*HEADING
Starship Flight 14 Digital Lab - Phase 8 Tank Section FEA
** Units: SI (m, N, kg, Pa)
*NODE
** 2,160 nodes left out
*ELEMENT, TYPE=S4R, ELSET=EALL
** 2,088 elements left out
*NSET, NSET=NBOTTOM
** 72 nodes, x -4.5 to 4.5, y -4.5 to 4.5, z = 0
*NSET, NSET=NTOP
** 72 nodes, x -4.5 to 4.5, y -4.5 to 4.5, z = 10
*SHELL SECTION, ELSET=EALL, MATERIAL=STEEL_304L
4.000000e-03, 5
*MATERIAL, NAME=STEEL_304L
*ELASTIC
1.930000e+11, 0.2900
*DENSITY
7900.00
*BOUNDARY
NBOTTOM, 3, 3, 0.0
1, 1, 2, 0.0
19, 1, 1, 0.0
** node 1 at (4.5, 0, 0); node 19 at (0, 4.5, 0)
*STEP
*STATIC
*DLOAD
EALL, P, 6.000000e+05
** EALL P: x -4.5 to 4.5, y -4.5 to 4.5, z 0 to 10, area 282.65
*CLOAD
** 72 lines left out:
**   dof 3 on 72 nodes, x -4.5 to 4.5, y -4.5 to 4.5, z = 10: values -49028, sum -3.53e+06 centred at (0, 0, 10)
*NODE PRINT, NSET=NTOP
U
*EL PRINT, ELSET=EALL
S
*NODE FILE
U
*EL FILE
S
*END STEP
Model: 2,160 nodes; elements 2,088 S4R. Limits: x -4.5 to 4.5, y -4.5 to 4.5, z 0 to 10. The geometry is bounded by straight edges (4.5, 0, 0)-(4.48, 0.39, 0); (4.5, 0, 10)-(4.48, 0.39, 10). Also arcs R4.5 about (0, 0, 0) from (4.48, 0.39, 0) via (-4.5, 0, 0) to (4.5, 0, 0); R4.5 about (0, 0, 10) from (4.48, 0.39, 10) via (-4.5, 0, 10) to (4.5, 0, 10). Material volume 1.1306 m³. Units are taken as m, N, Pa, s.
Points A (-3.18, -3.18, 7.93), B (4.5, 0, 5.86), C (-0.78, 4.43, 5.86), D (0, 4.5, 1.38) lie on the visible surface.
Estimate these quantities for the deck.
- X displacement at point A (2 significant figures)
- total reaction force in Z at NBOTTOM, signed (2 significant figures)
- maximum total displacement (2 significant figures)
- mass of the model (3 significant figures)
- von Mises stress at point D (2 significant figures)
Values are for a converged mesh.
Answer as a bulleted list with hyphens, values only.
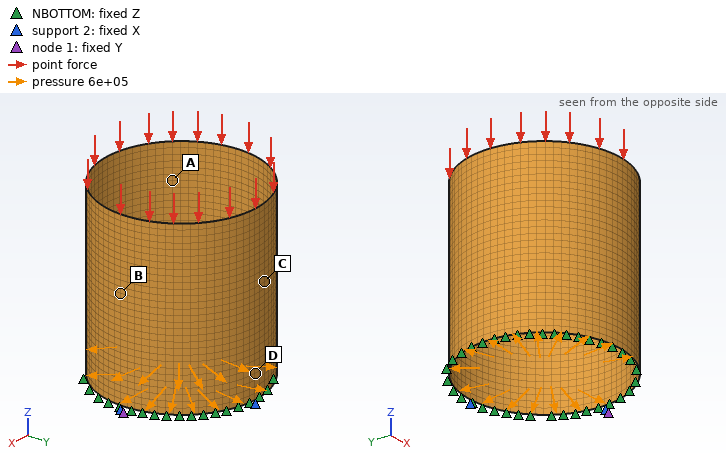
- -0.038 m
- 3.5e+06 N
- 0.047 m
- 8930 kg
- 6.9e+08 Pa
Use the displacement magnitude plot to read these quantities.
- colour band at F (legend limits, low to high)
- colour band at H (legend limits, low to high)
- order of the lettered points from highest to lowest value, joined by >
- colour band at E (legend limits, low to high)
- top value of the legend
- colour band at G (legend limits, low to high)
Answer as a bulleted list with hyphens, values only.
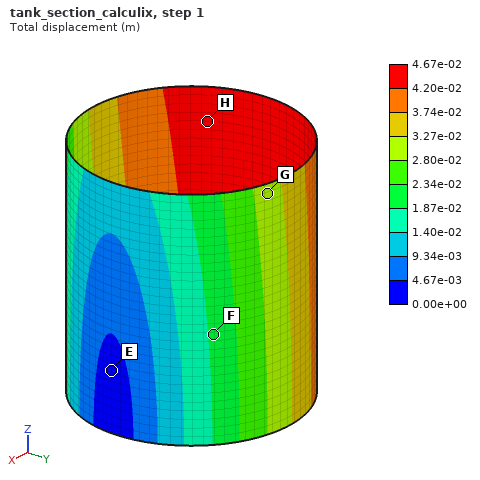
- 1.87e-02 to 2.34e-02 m
- 4.20e-02 to 4.67e-02 m
- H > G > F > E
- 0.00e+00 to 4.67e-03 m
- 4.67e-02 m
- 2.80e-02 to 3.27e-02 m
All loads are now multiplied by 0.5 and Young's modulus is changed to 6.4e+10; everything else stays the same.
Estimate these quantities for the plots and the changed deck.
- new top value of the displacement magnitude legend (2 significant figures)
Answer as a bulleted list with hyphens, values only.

- 0.070 m
